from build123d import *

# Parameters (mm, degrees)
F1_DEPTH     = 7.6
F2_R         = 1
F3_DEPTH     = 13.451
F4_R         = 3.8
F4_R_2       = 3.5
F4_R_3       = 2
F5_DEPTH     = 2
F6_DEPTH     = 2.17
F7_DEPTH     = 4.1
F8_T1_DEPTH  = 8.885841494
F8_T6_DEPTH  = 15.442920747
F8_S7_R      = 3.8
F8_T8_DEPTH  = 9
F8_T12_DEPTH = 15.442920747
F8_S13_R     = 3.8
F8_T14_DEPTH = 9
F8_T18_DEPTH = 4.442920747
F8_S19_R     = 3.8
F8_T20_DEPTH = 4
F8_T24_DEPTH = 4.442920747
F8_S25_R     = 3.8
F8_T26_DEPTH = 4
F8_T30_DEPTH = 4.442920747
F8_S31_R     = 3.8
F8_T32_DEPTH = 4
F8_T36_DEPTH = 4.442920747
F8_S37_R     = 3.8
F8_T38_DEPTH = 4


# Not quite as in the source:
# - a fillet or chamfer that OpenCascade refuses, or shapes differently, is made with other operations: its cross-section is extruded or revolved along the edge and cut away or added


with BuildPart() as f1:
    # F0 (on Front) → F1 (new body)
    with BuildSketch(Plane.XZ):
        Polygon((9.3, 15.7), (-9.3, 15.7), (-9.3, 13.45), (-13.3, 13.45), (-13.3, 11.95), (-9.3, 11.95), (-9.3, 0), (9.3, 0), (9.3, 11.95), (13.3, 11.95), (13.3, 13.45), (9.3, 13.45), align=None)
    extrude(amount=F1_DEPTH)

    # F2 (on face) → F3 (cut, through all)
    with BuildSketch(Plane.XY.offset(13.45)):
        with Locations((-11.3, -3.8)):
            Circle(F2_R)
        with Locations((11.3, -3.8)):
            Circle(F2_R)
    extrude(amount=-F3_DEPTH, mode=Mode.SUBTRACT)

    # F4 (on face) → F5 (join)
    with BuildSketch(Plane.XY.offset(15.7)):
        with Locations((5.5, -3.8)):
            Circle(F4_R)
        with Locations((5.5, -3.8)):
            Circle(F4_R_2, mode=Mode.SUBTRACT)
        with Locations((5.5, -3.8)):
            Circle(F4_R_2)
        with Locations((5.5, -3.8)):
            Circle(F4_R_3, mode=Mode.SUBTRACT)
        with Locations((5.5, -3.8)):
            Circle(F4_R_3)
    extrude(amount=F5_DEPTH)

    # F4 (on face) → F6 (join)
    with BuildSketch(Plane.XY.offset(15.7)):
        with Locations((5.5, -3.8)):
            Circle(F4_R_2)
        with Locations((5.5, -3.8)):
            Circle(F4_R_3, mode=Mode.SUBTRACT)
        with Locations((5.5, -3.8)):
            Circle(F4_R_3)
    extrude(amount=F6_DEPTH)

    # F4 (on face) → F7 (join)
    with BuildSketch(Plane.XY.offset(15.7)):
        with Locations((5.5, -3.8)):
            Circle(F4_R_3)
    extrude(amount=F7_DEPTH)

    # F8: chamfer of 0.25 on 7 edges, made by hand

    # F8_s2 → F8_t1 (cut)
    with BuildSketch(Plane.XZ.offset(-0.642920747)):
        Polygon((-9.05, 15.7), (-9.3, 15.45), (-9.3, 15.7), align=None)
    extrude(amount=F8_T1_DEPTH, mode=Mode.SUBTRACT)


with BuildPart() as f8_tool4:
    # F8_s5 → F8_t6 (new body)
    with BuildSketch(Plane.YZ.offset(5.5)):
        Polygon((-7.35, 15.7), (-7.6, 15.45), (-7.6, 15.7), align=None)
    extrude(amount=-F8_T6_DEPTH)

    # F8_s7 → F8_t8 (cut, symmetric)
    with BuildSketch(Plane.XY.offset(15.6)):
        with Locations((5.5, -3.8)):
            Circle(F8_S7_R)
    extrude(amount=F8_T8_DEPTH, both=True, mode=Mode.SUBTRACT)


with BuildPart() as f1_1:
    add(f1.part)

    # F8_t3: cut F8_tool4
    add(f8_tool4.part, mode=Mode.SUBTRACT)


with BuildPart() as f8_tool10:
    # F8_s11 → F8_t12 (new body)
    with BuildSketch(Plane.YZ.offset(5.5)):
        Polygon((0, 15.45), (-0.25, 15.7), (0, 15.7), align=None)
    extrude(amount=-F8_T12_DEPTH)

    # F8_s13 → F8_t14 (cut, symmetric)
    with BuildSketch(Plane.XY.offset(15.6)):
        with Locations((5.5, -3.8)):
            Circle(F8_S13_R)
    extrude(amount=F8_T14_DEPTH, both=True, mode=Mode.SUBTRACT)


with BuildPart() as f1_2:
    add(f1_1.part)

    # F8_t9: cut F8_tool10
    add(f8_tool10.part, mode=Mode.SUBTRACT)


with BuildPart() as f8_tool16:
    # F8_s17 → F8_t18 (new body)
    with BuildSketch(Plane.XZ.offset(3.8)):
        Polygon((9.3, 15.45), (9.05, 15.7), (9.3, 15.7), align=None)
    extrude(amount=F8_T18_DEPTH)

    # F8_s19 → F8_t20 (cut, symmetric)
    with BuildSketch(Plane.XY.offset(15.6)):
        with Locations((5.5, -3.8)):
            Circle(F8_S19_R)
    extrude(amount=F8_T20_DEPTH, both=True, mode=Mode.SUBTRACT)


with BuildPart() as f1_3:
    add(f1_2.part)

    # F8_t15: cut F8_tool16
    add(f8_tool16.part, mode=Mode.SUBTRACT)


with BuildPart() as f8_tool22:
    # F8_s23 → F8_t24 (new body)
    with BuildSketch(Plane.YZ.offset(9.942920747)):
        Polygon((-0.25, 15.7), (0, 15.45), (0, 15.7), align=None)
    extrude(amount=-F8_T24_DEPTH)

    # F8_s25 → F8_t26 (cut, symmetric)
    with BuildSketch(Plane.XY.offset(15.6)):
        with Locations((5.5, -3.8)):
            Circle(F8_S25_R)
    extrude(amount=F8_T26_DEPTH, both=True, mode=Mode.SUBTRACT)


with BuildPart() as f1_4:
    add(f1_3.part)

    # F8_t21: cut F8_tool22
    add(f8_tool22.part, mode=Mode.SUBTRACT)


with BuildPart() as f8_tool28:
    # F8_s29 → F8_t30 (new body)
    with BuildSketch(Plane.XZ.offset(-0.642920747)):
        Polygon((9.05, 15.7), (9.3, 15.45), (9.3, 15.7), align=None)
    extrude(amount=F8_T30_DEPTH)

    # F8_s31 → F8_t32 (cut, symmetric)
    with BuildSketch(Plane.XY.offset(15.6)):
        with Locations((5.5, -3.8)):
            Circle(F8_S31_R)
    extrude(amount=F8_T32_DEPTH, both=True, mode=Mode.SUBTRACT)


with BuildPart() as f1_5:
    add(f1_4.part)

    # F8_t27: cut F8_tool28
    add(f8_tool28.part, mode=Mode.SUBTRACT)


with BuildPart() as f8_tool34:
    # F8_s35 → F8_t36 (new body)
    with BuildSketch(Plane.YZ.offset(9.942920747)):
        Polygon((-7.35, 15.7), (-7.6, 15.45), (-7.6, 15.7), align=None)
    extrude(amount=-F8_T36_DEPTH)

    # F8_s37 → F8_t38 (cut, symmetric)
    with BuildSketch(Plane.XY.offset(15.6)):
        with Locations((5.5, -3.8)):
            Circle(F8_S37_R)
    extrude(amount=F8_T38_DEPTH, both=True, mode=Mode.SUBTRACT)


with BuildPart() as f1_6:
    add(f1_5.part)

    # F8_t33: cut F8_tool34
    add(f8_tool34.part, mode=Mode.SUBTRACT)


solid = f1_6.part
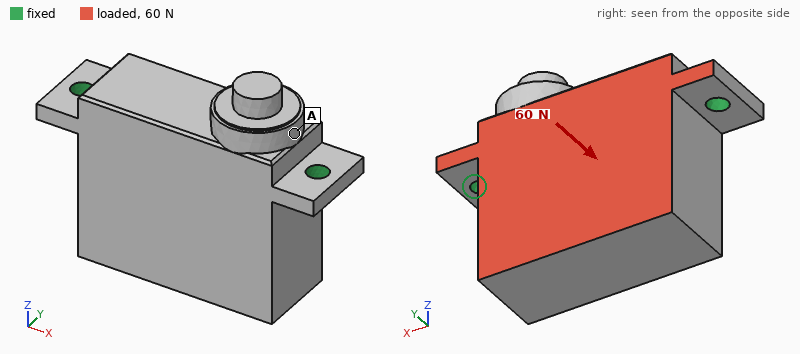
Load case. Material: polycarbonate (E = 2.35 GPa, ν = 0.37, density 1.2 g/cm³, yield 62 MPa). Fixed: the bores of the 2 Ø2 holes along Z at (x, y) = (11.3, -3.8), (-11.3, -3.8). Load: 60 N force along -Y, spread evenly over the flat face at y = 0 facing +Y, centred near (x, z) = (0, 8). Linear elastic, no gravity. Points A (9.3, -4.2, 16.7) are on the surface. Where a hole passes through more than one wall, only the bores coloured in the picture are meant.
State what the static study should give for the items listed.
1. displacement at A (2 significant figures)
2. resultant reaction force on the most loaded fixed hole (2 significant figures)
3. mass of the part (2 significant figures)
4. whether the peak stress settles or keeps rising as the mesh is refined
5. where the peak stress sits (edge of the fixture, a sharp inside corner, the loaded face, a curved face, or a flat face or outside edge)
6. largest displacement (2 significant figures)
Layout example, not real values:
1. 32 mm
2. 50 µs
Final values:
1. 0.095 mm
2. 30 N
3. 2.9 g
4. keeps rising
5. edge of the fixture
6. 0.38 mm
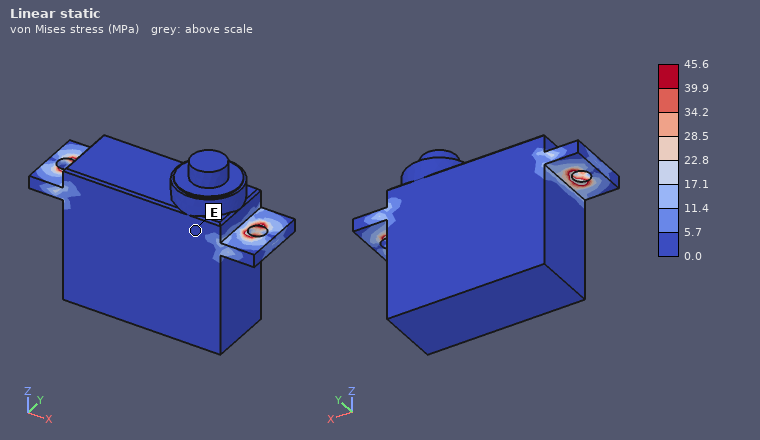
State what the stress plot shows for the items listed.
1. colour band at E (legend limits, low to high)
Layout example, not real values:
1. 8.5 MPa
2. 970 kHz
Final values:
1. 0.0 to 5.7 MPa
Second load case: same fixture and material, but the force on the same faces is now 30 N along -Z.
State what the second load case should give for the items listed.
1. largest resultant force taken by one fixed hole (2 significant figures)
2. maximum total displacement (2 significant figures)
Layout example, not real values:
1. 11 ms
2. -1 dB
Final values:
1. 15 N
2. 0.14 mm
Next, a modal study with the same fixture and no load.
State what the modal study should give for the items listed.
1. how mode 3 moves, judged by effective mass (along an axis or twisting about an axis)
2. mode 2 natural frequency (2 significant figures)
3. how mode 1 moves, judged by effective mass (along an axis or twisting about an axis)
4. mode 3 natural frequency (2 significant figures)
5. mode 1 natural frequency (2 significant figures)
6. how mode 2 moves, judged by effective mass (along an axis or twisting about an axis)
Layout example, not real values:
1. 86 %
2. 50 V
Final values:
1. along X
2. 5600 Hz
3. along Y
4. 6200 Hz
5. 1400 Hz
6. along Z
